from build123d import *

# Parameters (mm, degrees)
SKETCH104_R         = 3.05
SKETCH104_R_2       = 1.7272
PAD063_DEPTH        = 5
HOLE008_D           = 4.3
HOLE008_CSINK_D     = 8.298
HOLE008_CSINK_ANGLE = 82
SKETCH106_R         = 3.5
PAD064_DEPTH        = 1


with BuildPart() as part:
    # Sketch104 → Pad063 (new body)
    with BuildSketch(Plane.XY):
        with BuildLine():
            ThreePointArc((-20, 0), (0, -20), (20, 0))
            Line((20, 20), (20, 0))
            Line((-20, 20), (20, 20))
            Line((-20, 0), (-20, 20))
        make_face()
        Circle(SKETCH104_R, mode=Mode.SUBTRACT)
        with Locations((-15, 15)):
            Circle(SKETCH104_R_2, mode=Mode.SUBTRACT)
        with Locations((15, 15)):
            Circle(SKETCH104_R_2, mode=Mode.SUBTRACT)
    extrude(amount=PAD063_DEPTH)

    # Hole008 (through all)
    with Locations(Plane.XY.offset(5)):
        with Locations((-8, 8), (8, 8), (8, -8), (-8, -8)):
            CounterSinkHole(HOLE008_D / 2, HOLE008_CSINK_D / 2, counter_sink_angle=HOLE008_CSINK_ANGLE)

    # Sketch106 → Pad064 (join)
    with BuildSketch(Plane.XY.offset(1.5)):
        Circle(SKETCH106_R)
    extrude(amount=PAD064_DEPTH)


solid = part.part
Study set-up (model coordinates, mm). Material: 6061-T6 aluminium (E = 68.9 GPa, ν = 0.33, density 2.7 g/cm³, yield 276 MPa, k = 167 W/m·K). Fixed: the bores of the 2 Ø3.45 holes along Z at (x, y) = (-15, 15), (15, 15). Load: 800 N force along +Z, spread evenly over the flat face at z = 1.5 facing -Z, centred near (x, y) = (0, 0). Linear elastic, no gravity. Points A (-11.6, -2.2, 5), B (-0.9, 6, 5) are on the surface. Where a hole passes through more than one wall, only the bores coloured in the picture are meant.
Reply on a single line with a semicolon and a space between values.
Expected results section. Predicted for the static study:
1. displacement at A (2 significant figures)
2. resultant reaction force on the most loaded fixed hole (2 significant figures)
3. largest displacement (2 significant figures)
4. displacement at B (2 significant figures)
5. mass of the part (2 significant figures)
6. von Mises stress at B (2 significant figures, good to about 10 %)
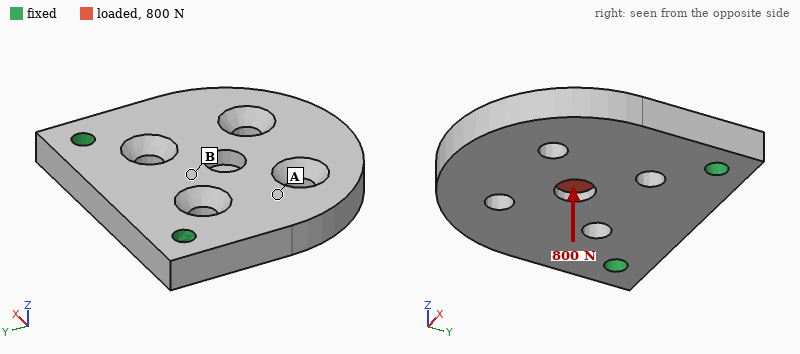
0.067 mm; 400 N; 0.16 mm; 0.042 mm; 17 g; 45 MPa
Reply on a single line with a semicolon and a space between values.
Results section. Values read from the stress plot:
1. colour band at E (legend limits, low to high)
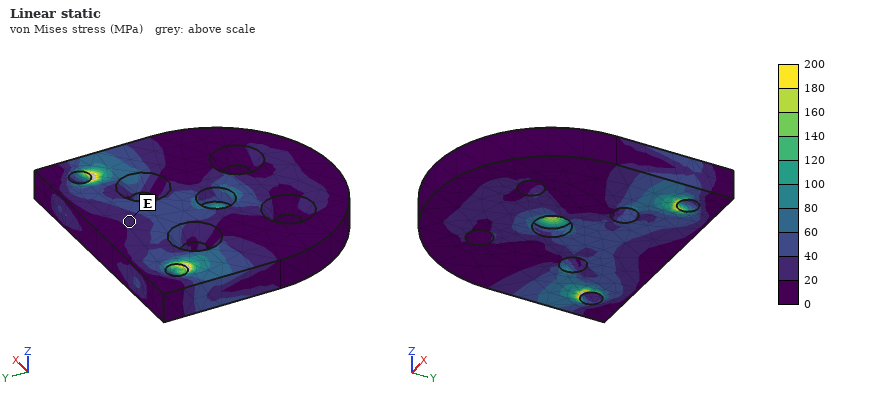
20 to 40 MPa
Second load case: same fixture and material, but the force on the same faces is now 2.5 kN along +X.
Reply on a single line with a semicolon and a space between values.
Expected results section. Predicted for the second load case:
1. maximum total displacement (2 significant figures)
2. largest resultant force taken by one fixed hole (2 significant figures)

22 µm; 1.7 kN
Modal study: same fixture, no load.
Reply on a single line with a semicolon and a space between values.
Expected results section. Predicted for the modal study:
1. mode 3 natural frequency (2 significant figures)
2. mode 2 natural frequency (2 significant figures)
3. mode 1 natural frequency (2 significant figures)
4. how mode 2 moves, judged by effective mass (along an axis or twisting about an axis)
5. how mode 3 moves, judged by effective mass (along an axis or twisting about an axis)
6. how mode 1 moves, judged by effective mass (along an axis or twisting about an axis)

17 kHz; 9300 Hz; 3400 Hz; twisting about Y; along X; along Z
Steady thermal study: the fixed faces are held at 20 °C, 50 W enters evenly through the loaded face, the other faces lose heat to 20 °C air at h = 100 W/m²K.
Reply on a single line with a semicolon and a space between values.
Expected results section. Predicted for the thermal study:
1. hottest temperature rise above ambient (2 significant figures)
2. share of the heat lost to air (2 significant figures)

69 K; 14 %
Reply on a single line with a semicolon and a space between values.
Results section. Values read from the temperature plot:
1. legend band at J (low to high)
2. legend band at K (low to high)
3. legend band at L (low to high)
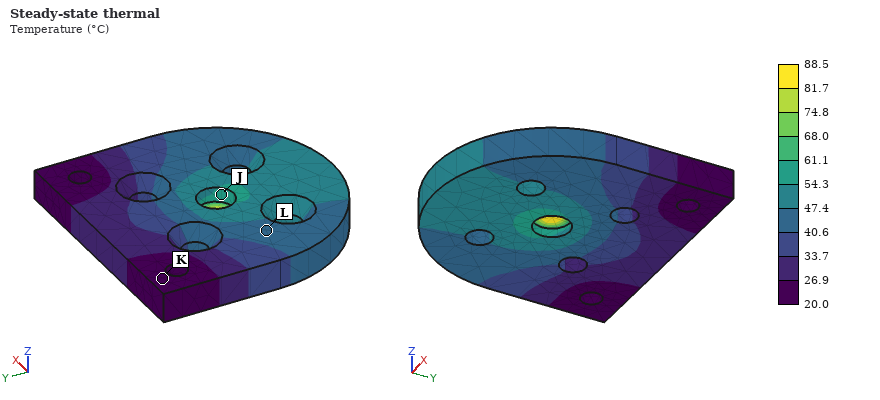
54.3 to 61.1 °C; 20.0 to 26.9 °C; 40.6 to 47.4 °C
